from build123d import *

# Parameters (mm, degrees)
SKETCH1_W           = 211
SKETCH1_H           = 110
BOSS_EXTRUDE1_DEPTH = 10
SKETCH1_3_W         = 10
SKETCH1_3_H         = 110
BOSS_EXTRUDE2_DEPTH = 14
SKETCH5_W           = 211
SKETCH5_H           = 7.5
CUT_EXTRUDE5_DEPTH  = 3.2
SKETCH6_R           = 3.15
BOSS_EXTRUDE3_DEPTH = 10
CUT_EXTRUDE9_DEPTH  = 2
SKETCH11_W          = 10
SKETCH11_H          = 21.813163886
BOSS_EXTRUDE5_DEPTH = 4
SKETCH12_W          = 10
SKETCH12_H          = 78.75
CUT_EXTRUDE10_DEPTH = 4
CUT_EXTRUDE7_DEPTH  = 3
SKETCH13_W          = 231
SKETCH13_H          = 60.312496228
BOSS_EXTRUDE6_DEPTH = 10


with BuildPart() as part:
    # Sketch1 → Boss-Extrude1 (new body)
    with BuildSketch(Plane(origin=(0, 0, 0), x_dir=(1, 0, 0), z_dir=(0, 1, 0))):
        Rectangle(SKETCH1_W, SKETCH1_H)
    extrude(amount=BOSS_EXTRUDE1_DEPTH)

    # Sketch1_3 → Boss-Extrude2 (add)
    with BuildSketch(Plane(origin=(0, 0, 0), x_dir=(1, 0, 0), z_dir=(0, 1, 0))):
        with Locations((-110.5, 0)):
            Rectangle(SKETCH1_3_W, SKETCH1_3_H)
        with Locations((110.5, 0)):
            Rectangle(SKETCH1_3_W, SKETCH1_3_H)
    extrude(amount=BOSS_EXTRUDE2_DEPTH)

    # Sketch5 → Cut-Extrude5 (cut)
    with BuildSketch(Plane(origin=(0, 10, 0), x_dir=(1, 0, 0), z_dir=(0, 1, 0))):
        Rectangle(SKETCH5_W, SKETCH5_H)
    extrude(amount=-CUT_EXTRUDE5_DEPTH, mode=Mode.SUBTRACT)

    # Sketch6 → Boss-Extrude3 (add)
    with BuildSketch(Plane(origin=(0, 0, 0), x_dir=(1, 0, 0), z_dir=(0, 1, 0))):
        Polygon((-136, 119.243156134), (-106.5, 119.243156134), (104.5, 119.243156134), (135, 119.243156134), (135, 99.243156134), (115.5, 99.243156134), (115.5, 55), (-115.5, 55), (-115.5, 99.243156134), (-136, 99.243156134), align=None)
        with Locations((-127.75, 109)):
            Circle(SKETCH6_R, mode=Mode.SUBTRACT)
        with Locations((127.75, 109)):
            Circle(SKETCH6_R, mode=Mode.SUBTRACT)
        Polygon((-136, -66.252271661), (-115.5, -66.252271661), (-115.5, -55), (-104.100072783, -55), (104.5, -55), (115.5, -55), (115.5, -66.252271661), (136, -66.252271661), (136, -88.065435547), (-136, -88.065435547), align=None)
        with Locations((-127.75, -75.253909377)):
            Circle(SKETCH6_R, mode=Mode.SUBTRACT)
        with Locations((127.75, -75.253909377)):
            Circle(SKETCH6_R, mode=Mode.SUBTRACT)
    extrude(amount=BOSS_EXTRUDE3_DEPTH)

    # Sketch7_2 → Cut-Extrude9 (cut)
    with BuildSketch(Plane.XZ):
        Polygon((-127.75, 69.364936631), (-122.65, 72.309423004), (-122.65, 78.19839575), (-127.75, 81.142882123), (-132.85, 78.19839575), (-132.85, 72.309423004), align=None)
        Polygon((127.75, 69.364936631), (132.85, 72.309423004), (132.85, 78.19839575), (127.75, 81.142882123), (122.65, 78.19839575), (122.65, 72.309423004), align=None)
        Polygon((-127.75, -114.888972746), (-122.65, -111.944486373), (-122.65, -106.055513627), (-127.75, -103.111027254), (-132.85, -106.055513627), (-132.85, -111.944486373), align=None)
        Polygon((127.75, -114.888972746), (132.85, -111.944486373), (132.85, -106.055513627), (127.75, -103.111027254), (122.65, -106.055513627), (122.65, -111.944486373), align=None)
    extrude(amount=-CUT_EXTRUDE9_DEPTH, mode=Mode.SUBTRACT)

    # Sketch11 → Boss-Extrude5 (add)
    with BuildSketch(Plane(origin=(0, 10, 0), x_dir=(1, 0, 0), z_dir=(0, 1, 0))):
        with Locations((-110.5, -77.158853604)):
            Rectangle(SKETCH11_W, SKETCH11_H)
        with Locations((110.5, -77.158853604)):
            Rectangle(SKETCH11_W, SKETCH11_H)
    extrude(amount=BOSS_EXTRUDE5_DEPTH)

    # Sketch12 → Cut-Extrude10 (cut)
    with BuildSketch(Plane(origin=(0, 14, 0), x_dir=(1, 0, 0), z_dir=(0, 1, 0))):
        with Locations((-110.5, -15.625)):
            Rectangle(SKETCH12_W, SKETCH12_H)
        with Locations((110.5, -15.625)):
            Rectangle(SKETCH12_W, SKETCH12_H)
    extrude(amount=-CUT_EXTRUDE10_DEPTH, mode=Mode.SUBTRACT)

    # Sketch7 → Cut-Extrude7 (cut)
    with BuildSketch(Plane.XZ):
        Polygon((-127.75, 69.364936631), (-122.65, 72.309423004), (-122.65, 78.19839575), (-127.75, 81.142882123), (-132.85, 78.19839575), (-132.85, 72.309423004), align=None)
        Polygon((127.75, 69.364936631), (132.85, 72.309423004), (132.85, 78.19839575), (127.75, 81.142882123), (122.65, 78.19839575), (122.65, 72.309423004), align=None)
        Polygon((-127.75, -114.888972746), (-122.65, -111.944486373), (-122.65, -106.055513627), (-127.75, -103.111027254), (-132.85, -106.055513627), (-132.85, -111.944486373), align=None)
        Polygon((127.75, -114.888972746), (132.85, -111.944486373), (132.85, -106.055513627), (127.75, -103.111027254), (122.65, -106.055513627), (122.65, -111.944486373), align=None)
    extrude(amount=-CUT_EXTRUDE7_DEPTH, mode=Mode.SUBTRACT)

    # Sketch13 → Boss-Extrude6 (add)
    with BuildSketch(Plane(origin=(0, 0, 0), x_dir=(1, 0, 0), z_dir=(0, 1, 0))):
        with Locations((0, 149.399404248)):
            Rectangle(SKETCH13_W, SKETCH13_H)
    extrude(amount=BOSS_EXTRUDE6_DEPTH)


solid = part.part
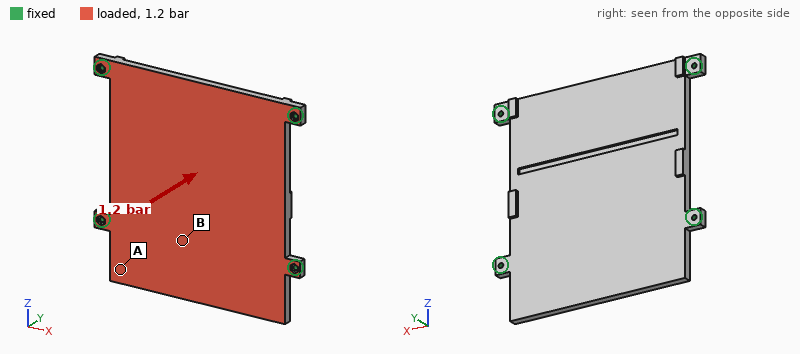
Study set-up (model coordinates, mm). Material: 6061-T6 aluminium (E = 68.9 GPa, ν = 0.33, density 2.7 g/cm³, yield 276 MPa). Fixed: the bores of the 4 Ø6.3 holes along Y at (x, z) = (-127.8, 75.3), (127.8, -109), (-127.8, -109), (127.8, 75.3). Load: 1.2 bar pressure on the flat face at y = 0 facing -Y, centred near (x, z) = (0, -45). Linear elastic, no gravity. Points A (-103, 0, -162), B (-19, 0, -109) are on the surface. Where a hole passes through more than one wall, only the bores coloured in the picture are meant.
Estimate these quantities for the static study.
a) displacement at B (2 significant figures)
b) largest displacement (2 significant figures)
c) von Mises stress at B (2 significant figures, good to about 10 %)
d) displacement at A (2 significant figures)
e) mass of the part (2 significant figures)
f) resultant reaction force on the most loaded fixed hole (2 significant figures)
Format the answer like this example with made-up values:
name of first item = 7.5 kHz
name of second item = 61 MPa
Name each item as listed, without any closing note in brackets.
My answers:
displacement at B = 0.63 mm
largest displacement = 0.79 mm
von Mises stress at B = 37 MPa
displacement at A = 0.27 mm
mass of the part = 1.7 kg
resultant reaction force on the most loaded fixed hole = 3.0 kN
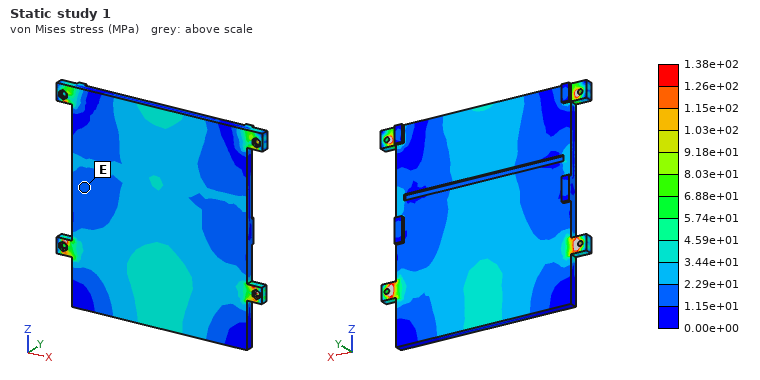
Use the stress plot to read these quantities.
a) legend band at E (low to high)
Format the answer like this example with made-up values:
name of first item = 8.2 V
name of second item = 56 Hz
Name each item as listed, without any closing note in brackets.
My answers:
legend band at E = 1.15e+01 to 2.29e+01 MPa
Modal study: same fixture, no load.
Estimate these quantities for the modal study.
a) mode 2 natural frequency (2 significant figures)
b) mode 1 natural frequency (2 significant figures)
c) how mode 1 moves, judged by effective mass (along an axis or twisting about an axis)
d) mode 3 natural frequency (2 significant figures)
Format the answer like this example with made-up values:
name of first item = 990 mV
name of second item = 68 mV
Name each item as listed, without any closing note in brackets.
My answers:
mode 2 natural frequency = 550 Hz
mode 1 natural frequency = 470 Hz
how mode 1 moves, judged by effective mass = along Y
mode 3 natural frequency = 1000 Hz
